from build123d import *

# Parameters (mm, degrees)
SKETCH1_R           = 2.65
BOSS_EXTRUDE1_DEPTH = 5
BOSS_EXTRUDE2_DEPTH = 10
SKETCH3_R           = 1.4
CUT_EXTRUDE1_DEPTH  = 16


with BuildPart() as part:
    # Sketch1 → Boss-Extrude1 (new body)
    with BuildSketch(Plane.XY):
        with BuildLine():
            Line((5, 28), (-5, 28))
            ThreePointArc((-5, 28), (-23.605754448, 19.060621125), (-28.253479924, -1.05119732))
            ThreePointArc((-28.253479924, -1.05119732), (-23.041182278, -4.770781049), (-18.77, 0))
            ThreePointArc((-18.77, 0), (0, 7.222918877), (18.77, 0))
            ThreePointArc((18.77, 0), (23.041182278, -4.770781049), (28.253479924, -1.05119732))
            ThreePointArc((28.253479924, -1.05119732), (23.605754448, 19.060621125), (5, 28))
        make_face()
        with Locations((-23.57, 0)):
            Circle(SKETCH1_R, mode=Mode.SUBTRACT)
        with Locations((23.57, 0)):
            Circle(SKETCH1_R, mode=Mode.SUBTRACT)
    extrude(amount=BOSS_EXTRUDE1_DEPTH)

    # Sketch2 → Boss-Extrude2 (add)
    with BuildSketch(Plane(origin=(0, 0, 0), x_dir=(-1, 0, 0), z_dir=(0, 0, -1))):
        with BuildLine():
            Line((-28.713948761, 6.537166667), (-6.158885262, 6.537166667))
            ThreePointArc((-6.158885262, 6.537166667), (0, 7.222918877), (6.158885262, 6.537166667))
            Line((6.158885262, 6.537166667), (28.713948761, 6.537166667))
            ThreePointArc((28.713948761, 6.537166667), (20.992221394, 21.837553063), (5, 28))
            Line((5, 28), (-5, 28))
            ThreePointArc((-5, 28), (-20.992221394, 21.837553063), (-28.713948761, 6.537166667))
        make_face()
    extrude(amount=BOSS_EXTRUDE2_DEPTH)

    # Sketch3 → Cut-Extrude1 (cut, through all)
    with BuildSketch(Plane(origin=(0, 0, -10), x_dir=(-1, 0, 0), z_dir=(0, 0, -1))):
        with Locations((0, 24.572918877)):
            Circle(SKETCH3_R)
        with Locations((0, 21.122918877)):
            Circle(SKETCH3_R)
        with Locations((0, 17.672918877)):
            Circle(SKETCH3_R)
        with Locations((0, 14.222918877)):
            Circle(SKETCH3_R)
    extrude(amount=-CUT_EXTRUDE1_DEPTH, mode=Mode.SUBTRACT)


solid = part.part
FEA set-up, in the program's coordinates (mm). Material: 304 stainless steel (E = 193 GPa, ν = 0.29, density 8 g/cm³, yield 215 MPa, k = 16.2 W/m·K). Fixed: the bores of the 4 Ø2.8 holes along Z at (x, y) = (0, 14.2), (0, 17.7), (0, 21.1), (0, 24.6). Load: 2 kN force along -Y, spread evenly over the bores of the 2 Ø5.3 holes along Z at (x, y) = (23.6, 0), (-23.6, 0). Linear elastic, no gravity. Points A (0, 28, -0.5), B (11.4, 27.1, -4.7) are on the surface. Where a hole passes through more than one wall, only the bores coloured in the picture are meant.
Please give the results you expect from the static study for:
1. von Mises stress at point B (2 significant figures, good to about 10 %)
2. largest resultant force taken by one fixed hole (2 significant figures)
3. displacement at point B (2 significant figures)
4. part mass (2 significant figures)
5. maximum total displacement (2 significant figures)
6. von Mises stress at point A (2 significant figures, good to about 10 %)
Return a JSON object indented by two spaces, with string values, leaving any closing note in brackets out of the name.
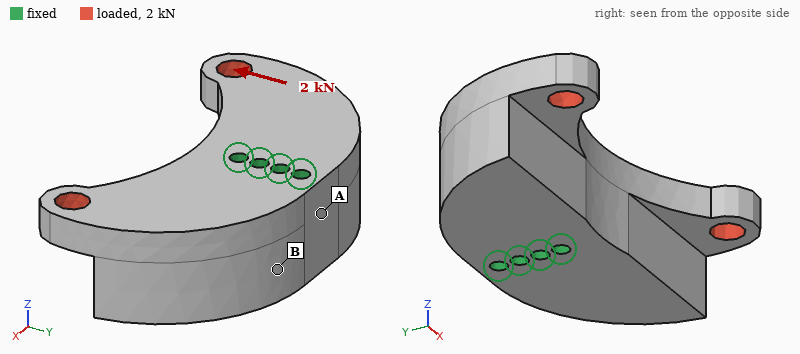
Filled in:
{
  "von Mises stress at point B": "11 MPa",
  "largest resultant force taken by one fixed hole": "750 N",
  "displacement at point B": "1.3 µm",
  "part mass": "120 g",
  "maximum total displacement": "8.9 µm",
  "von Mises stress at point A": "24 MPa"
}
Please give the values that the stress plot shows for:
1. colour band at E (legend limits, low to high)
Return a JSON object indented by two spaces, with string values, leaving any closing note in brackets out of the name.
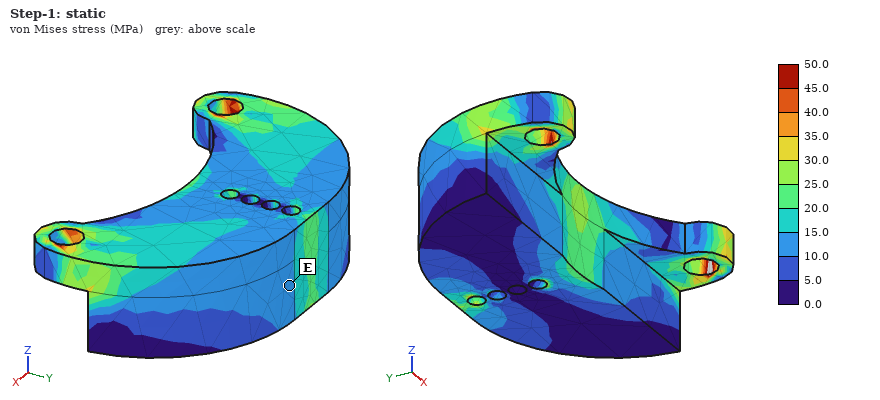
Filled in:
{
  "colour band at E": "10.0 to 15.0 MPa"
}
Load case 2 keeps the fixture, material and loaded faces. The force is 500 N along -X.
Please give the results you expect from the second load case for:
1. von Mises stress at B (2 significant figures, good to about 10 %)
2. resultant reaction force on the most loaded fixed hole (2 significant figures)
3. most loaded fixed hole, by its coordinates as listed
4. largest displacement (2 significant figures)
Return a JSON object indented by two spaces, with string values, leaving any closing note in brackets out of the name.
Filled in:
{
  "von Mises stress at B": "2.7 MPa",
  "resultant reaction force on the most loaded fixed hole": "950 N",
  "most loaded fixed hole, by its coordinates as listed": "(0, 14.2)",
  "largest displacement": "3.4 µm"
}
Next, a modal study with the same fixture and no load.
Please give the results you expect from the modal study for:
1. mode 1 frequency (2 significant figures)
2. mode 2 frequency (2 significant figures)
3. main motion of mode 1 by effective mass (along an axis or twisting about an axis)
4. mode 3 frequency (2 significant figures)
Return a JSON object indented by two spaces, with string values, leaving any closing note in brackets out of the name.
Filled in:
{
  "mode 1 frequency": "13 kHz",
  "mode 2 frequency": "14 kHz",
  "main motion of mode 1 by effective mass": "twisting about Y",
  "mode 3 frequency": "14 kHz"
}
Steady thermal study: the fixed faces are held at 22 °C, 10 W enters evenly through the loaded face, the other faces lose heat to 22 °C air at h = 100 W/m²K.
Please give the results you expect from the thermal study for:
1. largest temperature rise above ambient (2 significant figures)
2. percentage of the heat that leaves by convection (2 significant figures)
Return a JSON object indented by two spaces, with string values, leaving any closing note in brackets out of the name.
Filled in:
{
  "largest temperature rise above ambient": "66 K",
  "percentage of the heat that leaves by convection": "54 %"
}
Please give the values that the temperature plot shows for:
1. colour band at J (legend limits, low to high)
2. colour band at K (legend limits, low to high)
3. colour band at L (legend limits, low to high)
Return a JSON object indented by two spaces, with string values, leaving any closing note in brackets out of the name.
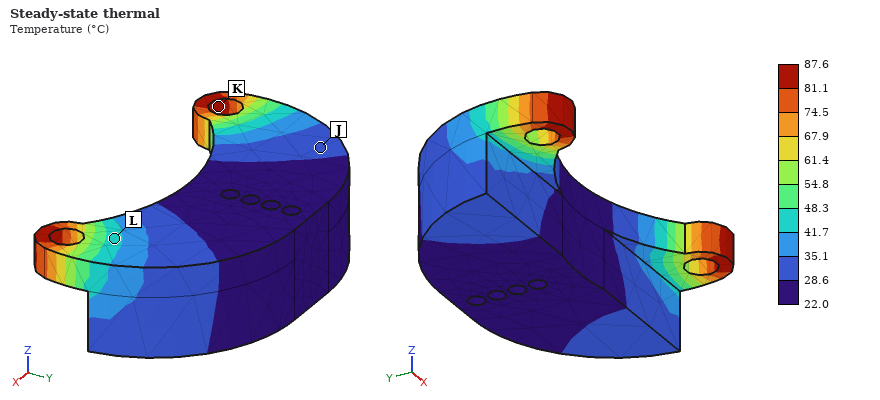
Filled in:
{
  "colour band at J": "28.6 to 35.1 °C",
  "colour band at K": "81.1 to 87.6 °C",
  "colour band at L": "41.7 to 48.3 °C"
}
